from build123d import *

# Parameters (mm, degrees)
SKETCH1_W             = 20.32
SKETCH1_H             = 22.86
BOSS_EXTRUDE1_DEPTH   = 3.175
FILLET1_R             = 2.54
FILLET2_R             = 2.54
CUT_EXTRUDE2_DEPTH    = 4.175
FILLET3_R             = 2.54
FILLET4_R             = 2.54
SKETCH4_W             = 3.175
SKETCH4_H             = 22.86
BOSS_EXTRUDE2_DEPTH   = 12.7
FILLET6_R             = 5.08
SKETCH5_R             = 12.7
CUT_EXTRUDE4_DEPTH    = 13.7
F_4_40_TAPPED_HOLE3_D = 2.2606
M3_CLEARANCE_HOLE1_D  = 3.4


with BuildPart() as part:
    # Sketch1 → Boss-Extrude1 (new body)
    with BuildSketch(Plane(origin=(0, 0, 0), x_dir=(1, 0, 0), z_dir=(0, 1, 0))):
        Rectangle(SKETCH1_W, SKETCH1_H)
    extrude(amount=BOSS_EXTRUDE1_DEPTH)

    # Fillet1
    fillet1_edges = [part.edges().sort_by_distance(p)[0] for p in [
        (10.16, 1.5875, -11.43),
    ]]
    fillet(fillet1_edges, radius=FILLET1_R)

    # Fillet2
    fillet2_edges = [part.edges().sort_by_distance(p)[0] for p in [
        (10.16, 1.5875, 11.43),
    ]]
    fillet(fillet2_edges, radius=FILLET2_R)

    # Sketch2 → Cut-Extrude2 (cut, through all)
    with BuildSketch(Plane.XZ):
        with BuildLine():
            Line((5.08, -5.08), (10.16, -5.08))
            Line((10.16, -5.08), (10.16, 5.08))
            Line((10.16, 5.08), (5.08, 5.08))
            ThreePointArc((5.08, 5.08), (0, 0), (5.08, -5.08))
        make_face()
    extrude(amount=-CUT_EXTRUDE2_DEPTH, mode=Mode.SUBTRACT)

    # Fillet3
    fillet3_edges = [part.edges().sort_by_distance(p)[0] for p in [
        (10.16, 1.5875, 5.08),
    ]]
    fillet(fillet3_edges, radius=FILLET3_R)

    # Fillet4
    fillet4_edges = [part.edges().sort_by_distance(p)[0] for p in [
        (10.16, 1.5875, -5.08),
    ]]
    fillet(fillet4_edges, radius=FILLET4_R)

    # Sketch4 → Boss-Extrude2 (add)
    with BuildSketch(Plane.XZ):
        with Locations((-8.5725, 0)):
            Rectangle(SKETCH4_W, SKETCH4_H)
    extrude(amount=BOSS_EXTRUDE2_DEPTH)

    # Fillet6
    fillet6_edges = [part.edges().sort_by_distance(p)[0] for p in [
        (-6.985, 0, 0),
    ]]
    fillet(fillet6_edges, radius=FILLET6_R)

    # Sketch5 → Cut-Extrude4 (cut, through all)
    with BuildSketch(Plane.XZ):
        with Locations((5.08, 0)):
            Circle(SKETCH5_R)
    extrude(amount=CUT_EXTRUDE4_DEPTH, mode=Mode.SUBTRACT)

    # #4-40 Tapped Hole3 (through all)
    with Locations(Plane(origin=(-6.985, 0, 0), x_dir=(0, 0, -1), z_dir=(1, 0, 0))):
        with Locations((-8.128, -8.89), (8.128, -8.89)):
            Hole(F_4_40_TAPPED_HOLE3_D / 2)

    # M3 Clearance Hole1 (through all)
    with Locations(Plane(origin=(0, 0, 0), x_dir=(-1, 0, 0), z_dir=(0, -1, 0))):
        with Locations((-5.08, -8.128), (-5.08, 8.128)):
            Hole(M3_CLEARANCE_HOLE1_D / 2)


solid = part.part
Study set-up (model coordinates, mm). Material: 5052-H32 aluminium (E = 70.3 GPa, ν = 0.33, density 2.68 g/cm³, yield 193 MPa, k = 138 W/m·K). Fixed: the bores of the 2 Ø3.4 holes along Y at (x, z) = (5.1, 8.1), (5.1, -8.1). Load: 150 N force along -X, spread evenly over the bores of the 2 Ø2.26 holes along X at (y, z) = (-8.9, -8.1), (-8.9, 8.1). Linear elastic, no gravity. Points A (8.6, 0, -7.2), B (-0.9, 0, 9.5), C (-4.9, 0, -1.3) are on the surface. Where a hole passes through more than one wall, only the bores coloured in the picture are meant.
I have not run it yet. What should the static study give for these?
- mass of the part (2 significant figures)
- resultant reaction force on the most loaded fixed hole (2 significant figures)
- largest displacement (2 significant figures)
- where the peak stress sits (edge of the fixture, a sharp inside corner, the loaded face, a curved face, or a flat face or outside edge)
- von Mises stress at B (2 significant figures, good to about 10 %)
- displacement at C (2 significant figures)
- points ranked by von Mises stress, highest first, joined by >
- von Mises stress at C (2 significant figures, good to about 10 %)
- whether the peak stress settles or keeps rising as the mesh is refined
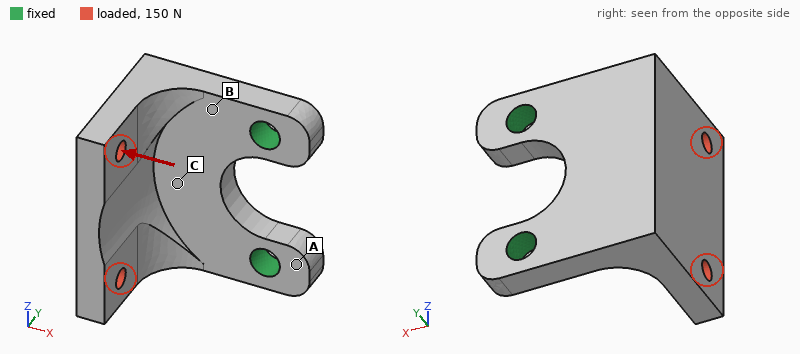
5.4 g
76 N
98 µm
edge of the fixture
59 MPa
24 µm
B > C > A
23 MPa
keeps rising
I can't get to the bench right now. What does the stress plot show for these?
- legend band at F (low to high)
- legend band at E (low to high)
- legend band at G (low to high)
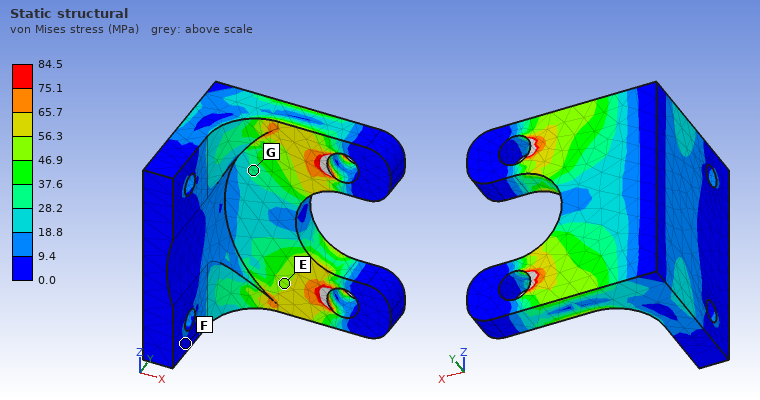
0.0 to 9.4 MPa
46.9 to 56.3 MPa
28.2 to 37.6 MPa
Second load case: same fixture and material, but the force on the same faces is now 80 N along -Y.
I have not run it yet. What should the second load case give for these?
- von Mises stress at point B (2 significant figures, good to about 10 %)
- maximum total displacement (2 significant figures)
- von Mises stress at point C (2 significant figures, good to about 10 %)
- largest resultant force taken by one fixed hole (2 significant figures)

22 MPa
37 µm
5.0 MPa
40 N
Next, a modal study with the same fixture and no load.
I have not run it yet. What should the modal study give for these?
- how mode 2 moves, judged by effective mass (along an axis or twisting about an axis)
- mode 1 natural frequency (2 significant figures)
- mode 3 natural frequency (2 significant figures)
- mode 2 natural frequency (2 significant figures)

along Z
4300 Hz
15 kHz
9100 Hz
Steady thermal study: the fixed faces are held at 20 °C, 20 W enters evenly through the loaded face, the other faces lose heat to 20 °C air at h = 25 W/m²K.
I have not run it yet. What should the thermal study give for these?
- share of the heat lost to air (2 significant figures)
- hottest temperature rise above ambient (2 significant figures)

5.3 %
51 K
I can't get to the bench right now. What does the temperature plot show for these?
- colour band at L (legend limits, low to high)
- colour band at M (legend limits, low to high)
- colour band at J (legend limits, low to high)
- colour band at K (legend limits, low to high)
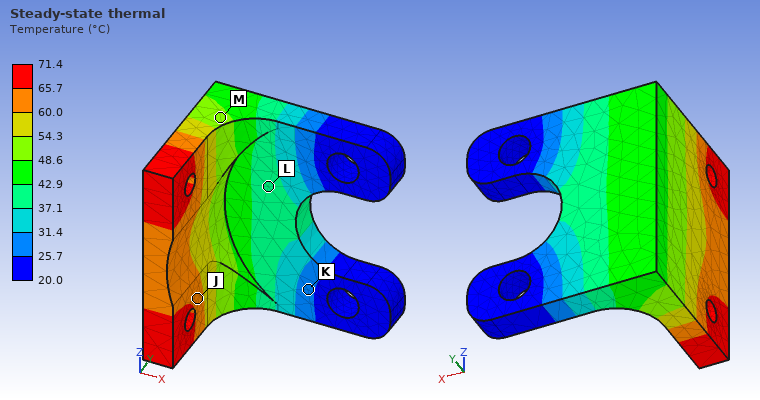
37.1 to 42.9 °C
48.6 to 54.3 °C
60.0 to 65.7 °C
25.7 to 31.4 °C
